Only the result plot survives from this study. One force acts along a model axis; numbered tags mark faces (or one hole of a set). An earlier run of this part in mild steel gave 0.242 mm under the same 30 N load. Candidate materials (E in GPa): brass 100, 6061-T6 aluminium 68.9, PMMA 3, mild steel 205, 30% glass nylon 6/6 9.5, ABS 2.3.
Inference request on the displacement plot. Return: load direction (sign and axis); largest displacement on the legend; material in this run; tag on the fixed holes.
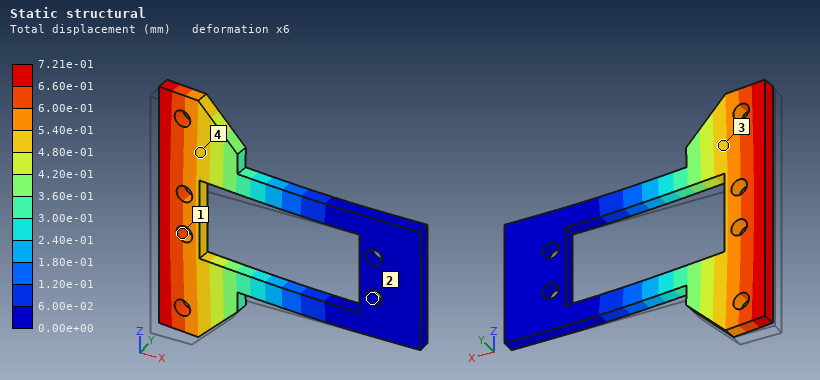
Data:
+Y
7.21e-01 mm
6061-T6 aluminium
2
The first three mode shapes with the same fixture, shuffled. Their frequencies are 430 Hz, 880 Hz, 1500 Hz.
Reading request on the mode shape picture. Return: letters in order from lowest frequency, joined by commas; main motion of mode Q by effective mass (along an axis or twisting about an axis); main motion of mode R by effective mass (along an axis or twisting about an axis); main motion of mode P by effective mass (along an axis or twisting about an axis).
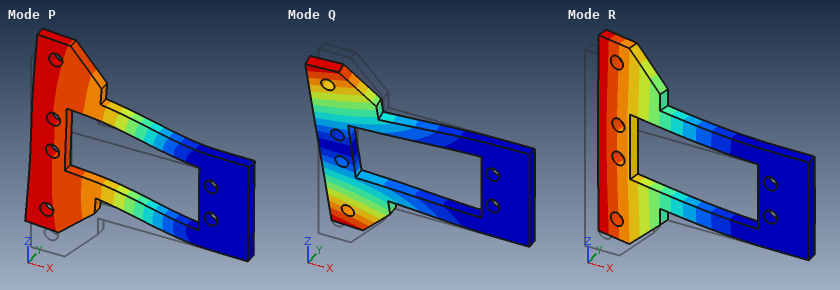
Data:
R, Q, P
twisting about X
along Y
along Z
